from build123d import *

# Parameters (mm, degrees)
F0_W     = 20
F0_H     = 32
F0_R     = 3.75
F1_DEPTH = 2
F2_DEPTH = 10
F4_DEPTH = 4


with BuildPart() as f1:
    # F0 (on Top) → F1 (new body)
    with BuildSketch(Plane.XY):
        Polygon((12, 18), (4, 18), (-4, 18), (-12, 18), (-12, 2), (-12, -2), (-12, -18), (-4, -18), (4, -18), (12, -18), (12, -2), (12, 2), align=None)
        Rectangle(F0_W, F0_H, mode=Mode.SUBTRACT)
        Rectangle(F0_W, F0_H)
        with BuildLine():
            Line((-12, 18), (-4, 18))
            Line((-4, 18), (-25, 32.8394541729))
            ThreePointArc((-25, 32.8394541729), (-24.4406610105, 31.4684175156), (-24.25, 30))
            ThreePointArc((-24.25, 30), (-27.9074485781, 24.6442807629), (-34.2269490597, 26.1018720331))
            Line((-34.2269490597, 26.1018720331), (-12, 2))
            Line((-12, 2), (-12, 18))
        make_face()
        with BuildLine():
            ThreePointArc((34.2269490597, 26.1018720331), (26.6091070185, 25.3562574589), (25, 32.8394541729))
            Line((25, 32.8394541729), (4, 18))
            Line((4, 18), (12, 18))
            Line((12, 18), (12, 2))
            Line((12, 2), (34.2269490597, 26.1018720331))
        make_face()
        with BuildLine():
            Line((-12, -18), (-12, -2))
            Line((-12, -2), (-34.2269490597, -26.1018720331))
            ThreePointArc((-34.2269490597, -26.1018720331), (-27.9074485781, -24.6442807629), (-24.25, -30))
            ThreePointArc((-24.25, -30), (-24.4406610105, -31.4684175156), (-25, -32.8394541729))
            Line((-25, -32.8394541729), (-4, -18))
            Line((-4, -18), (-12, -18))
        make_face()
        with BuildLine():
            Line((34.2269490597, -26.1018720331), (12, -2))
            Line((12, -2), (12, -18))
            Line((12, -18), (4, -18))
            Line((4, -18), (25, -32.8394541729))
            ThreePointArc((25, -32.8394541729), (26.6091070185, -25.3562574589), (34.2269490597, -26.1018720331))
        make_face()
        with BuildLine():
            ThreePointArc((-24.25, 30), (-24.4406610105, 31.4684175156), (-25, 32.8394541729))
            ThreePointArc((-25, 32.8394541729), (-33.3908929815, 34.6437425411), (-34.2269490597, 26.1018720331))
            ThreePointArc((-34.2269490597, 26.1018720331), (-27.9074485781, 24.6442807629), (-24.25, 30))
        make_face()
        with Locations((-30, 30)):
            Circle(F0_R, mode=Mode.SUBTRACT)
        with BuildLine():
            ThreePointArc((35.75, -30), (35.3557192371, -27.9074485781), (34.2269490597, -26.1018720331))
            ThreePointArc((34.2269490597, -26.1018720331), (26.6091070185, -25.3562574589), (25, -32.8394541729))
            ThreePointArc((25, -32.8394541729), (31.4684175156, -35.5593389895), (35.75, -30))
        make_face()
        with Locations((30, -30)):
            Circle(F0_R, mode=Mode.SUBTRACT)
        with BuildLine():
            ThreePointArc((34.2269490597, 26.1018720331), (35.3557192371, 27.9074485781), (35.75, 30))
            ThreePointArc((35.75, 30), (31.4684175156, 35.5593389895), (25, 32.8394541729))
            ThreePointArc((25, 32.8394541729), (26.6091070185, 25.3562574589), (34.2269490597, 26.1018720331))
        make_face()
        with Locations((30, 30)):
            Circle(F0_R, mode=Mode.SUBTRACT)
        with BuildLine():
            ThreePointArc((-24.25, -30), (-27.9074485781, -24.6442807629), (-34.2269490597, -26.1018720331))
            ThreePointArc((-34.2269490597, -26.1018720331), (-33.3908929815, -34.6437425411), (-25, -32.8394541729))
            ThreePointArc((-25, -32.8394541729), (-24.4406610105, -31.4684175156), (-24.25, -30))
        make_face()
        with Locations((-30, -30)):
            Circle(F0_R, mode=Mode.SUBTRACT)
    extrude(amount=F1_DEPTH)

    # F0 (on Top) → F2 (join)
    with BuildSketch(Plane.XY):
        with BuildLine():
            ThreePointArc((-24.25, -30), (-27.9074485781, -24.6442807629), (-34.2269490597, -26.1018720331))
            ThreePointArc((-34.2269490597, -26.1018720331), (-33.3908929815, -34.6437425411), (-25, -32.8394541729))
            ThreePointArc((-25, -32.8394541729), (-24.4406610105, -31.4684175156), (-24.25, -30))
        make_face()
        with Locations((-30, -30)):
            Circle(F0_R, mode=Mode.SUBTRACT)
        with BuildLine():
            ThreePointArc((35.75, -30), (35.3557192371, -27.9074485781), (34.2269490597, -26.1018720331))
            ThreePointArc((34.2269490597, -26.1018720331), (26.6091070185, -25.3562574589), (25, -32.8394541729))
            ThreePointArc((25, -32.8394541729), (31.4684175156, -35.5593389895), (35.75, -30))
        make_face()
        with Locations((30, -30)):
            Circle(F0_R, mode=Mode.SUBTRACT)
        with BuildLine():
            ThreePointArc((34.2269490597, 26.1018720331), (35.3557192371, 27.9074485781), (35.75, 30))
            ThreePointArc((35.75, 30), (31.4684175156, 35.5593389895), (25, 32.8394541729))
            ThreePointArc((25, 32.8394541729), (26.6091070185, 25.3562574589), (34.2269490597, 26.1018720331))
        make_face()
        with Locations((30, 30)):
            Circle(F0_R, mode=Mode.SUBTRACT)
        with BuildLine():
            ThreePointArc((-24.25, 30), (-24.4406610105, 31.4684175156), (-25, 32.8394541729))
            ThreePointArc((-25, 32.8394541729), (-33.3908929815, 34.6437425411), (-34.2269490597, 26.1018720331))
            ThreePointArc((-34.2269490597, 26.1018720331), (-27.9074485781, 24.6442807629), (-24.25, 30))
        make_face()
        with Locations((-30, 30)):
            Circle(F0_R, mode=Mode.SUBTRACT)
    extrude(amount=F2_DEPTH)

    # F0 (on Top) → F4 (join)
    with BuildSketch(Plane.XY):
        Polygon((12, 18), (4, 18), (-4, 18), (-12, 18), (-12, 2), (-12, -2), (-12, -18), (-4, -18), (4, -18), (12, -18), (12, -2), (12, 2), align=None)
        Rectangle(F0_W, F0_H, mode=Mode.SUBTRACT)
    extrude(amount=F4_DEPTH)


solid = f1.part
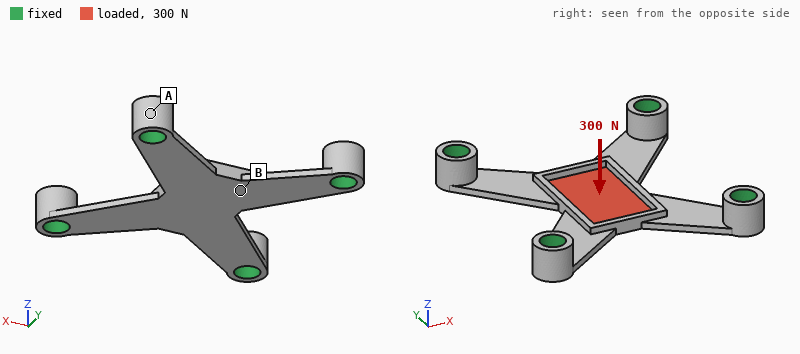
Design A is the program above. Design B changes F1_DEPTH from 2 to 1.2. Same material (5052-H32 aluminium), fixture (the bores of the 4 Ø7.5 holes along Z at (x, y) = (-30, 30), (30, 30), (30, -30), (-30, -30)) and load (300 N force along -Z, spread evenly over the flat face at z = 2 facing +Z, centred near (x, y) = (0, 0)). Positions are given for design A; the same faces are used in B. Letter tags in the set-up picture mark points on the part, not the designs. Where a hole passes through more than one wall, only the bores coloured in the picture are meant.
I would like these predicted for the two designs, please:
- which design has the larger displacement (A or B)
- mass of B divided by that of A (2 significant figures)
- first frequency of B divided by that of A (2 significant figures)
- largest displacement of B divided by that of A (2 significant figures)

B
0.79
0.72
2.4
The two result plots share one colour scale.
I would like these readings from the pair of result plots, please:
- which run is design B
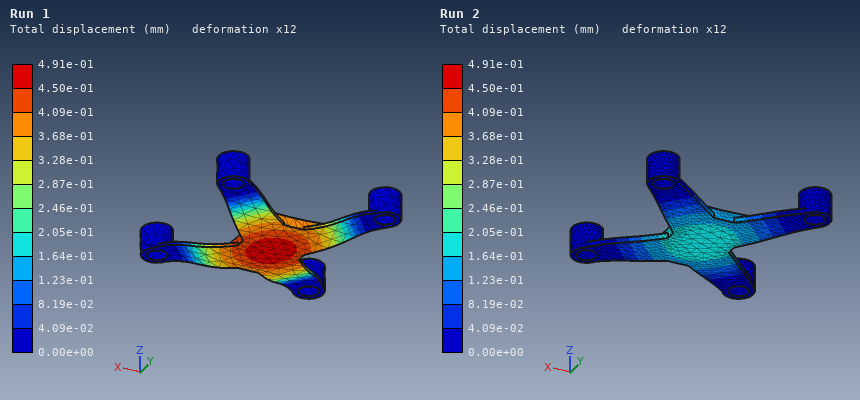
Run 1
